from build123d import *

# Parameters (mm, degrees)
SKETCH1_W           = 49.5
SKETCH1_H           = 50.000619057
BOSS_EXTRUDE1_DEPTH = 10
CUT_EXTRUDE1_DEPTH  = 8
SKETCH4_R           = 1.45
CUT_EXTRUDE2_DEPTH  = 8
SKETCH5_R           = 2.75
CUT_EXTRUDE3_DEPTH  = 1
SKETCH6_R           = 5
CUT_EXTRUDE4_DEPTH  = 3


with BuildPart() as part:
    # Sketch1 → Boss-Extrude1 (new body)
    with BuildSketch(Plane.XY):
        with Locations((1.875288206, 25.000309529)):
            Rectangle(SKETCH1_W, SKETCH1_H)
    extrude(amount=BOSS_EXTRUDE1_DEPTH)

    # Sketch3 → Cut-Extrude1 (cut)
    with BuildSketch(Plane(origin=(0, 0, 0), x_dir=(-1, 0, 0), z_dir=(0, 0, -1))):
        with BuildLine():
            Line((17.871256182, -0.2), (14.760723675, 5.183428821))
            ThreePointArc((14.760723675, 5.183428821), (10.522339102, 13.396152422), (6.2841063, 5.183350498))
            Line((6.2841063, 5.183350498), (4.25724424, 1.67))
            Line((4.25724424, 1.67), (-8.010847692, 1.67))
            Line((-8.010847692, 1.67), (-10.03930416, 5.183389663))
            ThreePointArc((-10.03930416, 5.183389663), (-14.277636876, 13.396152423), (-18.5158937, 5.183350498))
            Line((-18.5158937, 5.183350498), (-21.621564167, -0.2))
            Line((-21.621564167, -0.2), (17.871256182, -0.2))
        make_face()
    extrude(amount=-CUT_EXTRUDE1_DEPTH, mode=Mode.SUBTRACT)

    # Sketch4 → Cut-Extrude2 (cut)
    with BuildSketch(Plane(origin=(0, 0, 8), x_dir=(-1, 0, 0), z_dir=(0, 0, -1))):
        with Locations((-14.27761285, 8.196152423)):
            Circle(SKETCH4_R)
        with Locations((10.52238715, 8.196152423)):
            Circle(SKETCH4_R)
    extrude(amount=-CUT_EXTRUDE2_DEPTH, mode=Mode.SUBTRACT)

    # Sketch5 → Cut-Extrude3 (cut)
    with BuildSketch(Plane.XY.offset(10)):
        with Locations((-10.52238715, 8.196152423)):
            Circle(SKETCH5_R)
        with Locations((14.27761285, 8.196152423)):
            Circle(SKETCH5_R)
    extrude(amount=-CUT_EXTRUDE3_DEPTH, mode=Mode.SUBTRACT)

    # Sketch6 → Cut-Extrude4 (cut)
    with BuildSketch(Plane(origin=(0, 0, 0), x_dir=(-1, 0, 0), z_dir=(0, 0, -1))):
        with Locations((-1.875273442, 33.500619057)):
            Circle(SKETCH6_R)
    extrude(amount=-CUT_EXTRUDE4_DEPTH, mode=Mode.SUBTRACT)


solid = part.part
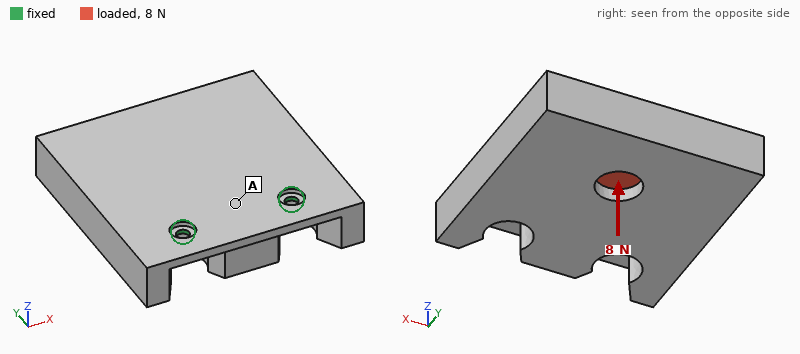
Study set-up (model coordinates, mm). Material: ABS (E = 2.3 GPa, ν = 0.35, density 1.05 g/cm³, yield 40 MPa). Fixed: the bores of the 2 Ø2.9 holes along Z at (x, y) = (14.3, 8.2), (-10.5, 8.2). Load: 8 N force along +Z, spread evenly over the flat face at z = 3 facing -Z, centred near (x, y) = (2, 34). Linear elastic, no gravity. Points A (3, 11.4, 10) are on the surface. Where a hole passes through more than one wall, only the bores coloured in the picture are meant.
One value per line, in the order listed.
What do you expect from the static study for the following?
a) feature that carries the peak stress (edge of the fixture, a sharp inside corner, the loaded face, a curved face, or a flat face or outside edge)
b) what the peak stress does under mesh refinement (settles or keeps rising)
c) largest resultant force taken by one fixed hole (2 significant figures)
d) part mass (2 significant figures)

edge of the fixture
keeps rising
4.0 N
23 g
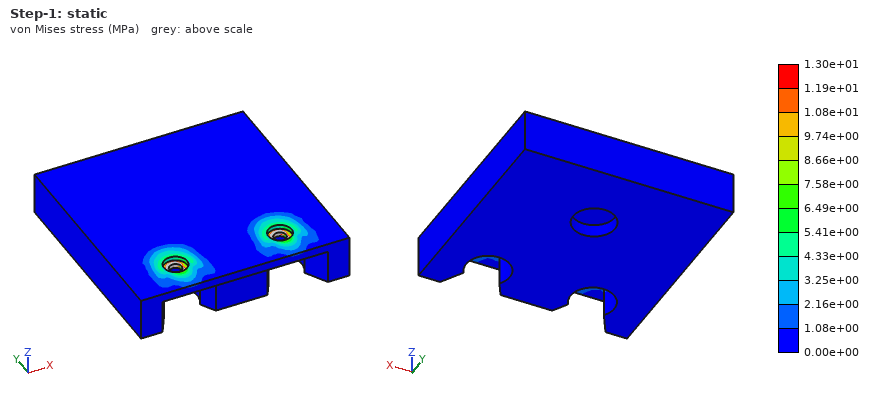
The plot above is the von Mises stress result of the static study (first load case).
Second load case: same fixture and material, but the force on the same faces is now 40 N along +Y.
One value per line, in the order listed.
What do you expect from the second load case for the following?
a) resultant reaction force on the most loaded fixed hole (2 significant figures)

20 N
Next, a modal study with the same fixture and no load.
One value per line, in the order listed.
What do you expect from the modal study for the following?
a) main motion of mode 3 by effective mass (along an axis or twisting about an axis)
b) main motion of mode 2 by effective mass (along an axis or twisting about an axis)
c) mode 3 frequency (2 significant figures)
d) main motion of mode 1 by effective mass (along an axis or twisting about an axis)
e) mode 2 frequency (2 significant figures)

along X
twisting about Y
1400 Hz
along Z
1100 Hz
